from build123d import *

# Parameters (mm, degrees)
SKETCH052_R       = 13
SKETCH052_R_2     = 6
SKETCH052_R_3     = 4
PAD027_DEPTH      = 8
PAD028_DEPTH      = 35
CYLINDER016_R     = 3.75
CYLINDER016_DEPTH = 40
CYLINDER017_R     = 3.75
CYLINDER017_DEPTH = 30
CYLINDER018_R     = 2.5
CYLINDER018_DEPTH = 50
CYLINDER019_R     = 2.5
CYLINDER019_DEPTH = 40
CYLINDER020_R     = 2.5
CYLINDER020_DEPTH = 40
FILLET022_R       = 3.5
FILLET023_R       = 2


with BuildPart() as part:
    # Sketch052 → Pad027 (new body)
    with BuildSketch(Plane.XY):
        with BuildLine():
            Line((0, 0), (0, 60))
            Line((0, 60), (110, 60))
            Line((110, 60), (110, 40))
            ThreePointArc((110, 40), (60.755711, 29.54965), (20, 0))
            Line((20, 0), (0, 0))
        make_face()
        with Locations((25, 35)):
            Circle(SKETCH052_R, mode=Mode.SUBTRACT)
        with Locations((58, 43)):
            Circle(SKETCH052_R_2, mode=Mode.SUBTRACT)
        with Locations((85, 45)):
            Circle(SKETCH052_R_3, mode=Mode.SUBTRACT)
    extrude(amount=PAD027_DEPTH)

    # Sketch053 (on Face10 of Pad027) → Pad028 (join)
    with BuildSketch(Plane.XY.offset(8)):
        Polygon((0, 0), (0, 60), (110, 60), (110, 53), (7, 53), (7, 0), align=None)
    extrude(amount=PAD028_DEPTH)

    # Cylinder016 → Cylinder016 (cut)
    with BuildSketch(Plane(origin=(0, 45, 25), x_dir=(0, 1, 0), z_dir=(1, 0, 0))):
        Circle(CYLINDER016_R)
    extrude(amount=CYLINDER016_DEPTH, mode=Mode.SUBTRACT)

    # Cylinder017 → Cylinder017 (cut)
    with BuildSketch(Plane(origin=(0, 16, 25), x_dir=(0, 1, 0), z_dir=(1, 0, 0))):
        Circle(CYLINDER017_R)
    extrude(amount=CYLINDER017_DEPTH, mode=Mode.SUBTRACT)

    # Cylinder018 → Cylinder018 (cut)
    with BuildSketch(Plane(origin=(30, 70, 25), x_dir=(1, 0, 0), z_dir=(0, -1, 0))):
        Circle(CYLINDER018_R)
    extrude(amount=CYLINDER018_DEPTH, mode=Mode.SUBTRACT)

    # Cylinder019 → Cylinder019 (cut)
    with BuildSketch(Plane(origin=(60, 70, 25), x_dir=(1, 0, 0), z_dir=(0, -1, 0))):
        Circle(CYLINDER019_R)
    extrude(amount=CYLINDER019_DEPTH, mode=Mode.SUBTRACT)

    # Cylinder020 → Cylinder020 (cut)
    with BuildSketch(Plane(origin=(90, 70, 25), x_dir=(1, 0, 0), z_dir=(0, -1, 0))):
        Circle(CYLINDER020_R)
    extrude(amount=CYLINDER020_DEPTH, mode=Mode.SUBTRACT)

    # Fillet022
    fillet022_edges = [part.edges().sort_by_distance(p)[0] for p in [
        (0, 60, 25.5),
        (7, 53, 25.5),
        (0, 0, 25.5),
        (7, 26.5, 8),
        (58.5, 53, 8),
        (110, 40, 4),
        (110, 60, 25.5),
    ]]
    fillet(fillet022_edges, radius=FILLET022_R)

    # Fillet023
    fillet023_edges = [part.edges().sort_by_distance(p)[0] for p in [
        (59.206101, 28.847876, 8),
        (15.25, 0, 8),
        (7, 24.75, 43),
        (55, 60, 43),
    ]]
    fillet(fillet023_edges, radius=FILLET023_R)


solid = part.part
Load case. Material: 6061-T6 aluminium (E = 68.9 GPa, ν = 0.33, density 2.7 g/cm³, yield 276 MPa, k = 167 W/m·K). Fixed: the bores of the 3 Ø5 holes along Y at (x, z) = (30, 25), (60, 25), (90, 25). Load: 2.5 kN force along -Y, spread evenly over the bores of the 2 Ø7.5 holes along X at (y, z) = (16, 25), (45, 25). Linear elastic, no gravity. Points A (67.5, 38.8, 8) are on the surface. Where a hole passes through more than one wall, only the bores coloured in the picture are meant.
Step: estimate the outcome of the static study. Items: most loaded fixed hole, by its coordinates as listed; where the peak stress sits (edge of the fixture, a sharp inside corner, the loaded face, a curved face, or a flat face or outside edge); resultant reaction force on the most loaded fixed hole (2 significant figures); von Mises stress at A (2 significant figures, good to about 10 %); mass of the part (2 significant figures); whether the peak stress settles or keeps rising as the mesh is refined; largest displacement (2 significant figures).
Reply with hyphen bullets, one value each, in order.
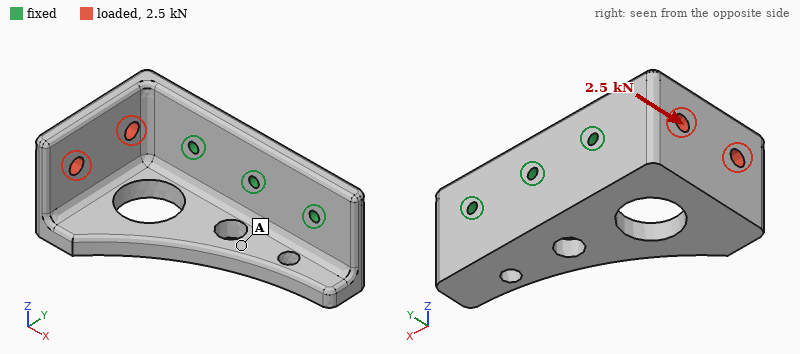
- (30, 25)
- edge of the fixture
- 3.4 kN
- 14 MPa
- 180 g
- keeps rising
- 0.17 mm
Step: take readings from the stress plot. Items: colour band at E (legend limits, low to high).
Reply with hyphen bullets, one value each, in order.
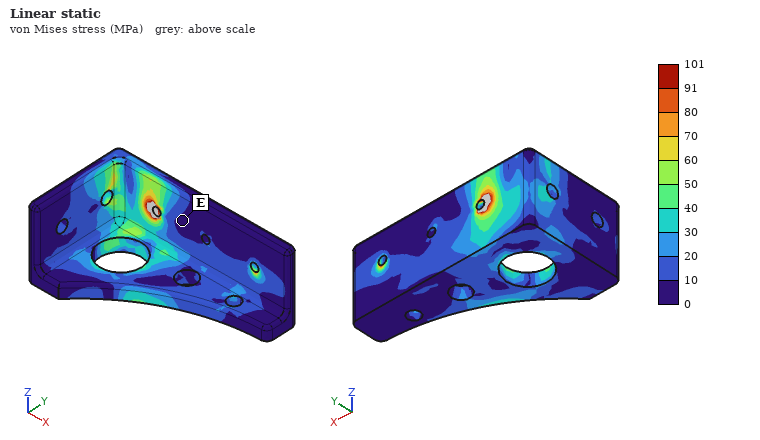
- 0 to 10 MPa
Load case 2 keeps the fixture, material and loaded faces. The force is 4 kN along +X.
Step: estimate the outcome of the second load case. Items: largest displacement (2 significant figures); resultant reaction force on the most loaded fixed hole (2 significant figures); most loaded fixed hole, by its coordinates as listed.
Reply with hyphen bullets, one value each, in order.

- 0.48 mm
- 2.8 kN
- (30, 25)
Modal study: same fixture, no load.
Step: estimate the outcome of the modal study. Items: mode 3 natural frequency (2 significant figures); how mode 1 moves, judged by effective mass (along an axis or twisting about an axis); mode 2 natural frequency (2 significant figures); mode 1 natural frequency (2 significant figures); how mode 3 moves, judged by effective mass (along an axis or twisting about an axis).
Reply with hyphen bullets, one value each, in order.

- 4000 Hz
- along Z
- 2400 Hz
- 1400 Hz
- along Y
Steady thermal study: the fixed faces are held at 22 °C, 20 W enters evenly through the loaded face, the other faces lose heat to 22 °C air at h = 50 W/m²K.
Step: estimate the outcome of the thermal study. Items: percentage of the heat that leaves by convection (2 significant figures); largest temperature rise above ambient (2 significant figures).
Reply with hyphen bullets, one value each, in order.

- 24 %
- 14 K
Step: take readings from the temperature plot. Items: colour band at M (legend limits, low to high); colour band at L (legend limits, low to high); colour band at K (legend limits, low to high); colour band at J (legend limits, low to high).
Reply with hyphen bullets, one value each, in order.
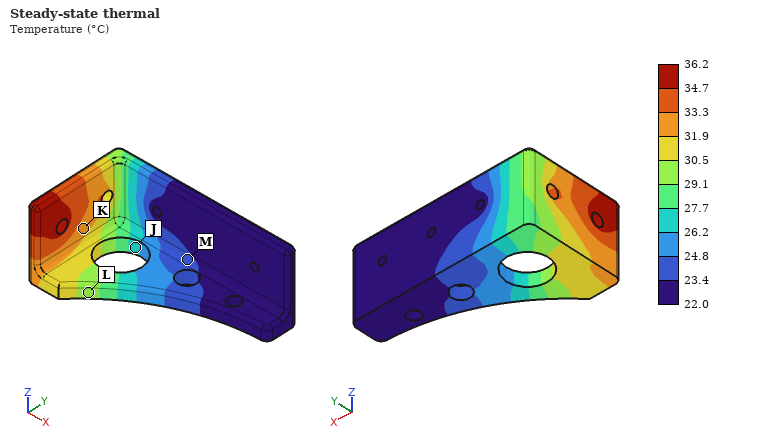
- 23.4 to 24.8 °C
- 29.1 to 30.5 °C
- 31.9 to 33.3 °C
- 26.2 to 27.7 °C
